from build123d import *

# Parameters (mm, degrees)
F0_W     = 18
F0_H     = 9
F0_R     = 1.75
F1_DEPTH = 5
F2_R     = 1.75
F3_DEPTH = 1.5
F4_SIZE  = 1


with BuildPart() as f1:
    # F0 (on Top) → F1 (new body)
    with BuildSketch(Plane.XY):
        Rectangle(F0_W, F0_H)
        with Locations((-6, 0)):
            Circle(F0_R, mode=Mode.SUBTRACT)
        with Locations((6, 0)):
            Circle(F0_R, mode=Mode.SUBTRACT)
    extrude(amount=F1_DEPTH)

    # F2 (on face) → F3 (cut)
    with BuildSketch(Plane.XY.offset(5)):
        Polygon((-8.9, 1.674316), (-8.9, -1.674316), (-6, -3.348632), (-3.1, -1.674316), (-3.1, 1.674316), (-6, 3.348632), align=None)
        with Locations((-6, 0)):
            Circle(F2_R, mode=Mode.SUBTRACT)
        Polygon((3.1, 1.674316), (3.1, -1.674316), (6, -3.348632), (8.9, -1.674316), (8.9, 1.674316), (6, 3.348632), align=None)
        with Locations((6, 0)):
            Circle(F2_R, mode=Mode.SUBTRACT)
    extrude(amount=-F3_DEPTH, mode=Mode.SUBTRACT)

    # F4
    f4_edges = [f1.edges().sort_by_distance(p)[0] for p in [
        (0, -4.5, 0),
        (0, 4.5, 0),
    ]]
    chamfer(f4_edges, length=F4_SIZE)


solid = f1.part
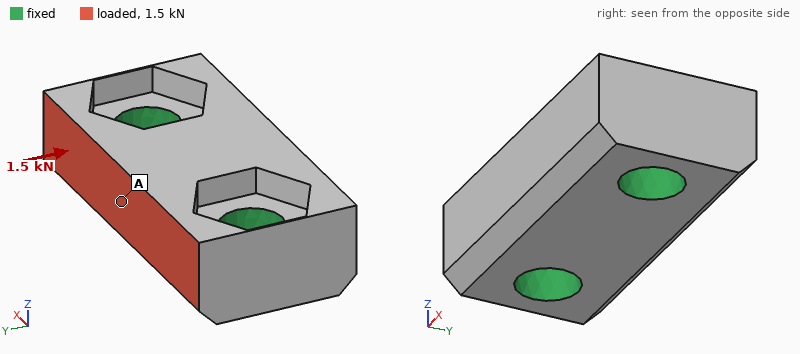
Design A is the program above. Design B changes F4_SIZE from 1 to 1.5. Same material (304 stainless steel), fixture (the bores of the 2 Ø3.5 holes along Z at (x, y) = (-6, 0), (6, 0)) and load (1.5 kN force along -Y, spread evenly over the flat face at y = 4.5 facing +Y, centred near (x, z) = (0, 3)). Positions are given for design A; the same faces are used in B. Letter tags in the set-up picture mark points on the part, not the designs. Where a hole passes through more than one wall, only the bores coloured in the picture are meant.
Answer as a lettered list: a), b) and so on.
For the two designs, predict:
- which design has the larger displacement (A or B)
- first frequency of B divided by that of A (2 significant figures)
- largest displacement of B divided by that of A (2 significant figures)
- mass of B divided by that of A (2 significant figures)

a) B
b) 1.0
c) 1.2
d) 0.96
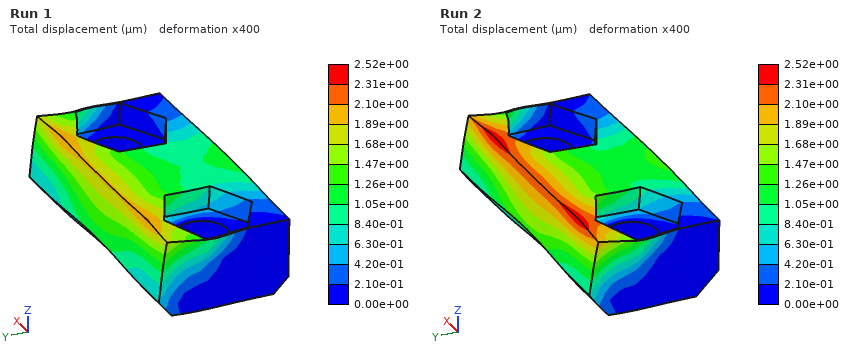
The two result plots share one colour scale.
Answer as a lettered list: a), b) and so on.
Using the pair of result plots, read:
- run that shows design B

a) Run 2
